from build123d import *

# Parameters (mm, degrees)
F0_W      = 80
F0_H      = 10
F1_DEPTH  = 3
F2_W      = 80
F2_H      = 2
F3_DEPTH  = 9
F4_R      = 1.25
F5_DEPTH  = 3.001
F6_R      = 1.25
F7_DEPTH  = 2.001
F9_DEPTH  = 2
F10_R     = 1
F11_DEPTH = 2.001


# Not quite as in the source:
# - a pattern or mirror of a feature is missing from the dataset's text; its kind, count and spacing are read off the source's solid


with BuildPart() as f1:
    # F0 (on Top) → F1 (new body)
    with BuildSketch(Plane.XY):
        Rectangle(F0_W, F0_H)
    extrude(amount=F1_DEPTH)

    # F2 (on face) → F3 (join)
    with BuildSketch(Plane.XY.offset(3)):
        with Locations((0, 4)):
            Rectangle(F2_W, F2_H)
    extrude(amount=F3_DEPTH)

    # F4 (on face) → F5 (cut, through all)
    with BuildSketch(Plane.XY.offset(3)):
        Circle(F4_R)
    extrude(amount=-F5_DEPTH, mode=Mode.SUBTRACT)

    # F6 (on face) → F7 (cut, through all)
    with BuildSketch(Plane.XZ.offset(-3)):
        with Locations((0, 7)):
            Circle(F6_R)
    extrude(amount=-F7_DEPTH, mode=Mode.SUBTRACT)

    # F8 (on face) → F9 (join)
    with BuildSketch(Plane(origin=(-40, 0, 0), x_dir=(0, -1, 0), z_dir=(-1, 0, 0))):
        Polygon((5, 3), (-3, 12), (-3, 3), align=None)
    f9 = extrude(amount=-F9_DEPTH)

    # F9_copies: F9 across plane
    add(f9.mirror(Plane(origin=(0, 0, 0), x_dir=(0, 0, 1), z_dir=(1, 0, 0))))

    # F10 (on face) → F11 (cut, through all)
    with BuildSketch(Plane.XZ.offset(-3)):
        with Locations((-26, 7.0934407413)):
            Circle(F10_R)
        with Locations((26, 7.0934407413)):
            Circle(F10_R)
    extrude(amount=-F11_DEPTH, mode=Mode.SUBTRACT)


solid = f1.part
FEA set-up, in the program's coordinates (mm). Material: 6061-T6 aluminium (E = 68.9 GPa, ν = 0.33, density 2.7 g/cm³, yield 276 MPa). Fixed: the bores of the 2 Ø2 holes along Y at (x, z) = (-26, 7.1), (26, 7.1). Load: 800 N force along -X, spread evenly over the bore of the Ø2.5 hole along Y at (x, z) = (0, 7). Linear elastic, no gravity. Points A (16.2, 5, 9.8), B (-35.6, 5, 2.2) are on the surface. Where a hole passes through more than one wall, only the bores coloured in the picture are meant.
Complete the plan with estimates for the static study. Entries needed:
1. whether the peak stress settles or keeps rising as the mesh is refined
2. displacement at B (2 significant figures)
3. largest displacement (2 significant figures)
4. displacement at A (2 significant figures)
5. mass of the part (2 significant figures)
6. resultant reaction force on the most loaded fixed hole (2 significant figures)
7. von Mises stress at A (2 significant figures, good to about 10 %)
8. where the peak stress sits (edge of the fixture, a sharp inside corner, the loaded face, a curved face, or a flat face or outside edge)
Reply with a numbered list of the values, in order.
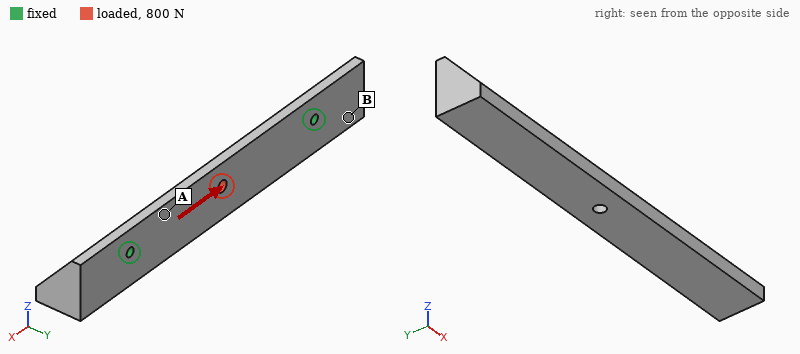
1. keeps rising
2. 3.8 µm
3. 8.7 µm
4. 3.3 µm
5. 11 g
6. 400 N
7. 22 MPa
8. edge of the fixture
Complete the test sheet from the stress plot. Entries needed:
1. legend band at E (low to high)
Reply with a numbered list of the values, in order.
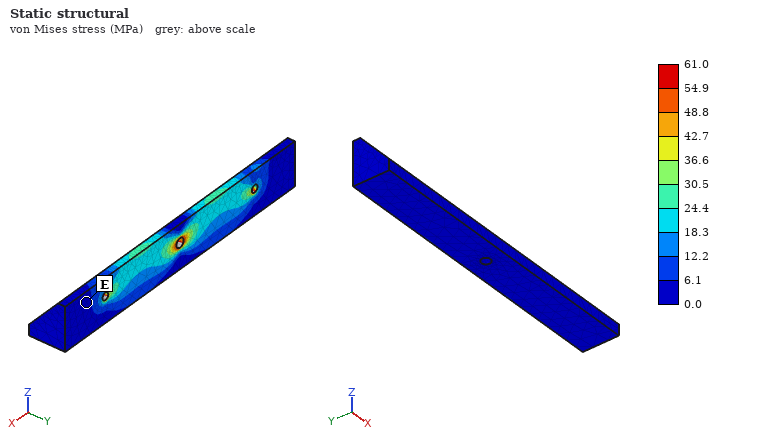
1. 0.0 to 6.1 MPa
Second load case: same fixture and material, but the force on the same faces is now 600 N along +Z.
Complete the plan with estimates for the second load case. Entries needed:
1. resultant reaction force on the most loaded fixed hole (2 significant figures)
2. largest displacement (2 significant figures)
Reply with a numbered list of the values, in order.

1. 410 N
2. 63 µm
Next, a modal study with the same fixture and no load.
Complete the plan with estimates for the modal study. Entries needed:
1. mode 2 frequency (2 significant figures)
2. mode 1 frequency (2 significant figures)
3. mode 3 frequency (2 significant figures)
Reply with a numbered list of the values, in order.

1. 6800 Hz
2. 5000 Hz
3. 7400 Hz
